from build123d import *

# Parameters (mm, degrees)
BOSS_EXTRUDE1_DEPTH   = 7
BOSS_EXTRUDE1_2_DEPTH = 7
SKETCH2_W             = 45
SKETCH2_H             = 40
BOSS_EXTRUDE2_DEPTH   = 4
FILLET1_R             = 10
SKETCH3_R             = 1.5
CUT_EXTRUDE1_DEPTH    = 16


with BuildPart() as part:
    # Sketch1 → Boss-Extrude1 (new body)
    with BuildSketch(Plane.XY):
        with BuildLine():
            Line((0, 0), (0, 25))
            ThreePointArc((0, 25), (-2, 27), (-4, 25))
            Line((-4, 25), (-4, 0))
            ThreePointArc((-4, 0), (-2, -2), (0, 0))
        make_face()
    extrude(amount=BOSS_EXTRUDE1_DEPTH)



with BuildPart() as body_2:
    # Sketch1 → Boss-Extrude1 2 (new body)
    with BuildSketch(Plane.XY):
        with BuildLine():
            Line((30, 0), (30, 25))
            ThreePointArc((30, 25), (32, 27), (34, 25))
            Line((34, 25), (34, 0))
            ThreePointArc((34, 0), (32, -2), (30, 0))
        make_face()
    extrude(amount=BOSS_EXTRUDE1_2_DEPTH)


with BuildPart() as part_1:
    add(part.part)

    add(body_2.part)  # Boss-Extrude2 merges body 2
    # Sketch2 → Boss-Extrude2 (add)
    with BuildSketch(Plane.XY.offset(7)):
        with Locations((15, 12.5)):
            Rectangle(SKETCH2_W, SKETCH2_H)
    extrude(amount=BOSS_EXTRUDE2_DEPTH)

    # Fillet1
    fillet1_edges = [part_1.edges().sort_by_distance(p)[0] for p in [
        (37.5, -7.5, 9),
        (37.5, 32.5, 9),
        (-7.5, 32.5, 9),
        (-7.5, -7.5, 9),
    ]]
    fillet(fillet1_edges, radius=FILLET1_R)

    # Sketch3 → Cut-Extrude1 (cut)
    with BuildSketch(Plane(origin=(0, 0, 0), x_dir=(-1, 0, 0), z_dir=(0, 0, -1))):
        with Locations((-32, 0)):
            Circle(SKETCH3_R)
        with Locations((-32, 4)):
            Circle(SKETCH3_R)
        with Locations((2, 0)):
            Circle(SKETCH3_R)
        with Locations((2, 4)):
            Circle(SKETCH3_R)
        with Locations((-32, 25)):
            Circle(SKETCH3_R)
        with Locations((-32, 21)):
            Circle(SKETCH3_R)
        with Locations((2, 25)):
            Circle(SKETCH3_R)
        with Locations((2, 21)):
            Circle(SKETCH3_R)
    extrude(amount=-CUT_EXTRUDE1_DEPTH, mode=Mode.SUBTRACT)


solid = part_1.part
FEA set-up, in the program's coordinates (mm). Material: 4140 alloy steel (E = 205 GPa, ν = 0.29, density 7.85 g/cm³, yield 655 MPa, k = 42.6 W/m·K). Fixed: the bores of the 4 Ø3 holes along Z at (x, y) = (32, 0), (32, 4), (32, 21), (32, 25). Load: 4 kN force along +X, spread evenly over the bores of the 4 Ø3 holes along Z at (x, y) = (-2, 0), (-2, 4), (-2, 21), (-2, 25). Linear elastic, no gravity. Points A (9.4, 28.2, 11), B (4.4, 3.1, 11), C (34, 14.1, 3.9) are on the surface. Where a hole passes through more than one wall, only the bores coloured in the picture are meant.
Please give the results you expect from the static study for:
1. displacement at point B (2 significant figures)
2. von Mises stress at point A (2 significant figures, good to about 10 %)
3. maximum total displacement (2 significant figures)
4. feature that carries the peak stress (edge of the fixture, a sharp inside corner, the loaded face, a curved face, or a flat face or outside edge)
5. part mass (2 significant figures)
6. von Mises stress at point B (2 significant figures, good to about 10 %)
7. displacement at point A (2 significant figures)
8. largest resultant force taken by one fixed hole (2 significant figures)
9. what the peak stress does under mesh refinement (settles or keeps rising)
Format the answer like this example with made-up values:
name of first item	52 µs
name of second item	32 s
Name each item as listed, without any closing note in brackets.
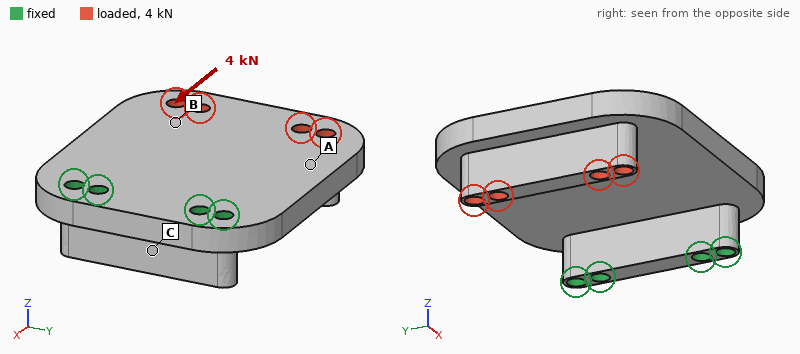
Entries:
displacement at point B	0.11 mm
von Mises stress at point A	100 MPa
maximum total displacement	0.23 mm
feature that carries the peak stress	a sharp inside corner
part mass	61 g
von Mises stress at point B	90 MPa
displacement at point A	0.074 mm
largest resultant force taken by one fixed hole	1.1 kN
what the peak stress does under mesh refinement	keeps rising
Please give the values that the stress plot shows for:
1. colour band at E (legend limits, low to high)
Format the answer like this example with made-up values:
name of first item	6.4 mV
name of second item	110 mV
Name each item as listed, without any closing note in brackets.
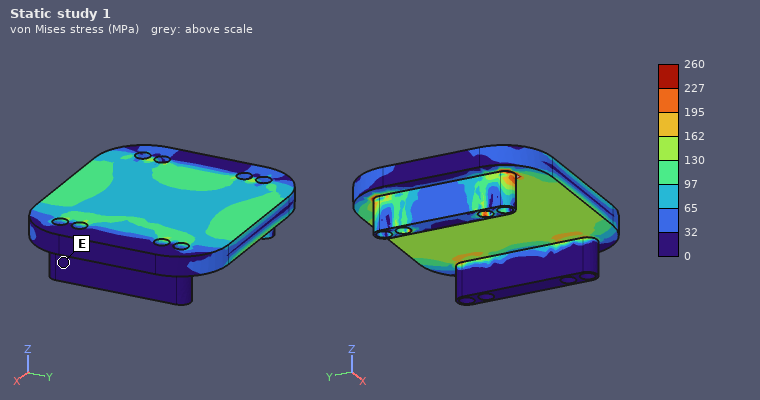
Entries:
colour band at E	0 to 32 MPa
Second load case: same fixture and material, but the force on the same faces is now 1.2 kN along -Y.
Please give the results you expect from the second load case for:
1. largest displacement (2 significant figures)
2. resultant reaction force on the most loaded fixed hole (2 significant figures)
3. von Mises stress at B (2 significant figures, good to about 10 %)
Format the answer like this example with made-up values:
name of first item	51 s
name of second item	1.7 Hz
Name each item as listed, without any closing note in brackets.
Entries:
largest displacement	32 µm
resultant reaction force on the most loaded fixed hole	1.3 kN
von Mises stress at B	13 MPa
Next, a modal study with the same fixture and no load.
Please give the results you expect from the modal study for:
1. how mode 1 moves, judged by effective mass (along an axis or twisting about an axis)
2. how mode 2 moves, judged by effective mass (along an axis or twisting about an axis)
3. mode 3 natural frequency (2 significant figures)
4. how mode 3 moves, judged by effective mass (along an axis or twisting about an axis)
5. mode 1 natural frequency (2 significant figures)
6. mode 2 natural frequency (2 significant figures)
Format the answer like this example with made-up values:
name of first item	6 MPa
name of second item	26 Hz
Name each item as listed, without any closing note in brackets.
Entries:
how mode 1 moves, judged by effective mass	along Z
how mode 2 moves, judged by effective mass	twisting about X
mode 3 natural frequency	12 kHz
how mode 3 moves, judged by effective mass	along Y
mode 1 natural frequency	2100 Hz
mode 2 natural frequency	5200 Hz
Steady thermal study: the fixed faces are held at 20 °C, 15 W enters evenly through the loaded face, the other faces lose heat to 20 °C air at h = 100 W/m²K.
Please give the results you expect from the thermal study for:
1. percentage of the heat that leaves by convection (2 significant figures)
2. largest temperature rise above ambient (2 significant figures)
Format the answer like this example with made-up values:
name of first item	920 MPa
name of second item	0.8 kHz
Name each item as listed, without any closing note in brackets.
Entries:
percentage of the heat that leaves by convection	60 %
largest temperature rise above ambient	60 K
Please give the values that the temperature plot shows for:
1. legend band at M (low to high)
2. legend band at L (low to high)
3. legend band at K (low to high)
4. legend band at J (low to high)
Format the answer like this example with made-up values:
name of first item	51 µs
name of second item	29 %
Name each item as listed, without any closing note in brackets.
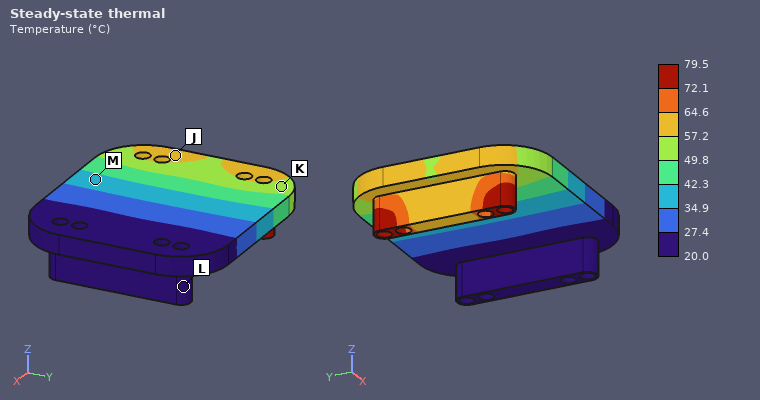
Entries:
legend band at M	34.9 to 42.3 °C
legend band at L	20.0 to 27.4 °C
legend band at K	49.8 to 57.2 °C
legend band at J	57.2 to 64.6 °C
